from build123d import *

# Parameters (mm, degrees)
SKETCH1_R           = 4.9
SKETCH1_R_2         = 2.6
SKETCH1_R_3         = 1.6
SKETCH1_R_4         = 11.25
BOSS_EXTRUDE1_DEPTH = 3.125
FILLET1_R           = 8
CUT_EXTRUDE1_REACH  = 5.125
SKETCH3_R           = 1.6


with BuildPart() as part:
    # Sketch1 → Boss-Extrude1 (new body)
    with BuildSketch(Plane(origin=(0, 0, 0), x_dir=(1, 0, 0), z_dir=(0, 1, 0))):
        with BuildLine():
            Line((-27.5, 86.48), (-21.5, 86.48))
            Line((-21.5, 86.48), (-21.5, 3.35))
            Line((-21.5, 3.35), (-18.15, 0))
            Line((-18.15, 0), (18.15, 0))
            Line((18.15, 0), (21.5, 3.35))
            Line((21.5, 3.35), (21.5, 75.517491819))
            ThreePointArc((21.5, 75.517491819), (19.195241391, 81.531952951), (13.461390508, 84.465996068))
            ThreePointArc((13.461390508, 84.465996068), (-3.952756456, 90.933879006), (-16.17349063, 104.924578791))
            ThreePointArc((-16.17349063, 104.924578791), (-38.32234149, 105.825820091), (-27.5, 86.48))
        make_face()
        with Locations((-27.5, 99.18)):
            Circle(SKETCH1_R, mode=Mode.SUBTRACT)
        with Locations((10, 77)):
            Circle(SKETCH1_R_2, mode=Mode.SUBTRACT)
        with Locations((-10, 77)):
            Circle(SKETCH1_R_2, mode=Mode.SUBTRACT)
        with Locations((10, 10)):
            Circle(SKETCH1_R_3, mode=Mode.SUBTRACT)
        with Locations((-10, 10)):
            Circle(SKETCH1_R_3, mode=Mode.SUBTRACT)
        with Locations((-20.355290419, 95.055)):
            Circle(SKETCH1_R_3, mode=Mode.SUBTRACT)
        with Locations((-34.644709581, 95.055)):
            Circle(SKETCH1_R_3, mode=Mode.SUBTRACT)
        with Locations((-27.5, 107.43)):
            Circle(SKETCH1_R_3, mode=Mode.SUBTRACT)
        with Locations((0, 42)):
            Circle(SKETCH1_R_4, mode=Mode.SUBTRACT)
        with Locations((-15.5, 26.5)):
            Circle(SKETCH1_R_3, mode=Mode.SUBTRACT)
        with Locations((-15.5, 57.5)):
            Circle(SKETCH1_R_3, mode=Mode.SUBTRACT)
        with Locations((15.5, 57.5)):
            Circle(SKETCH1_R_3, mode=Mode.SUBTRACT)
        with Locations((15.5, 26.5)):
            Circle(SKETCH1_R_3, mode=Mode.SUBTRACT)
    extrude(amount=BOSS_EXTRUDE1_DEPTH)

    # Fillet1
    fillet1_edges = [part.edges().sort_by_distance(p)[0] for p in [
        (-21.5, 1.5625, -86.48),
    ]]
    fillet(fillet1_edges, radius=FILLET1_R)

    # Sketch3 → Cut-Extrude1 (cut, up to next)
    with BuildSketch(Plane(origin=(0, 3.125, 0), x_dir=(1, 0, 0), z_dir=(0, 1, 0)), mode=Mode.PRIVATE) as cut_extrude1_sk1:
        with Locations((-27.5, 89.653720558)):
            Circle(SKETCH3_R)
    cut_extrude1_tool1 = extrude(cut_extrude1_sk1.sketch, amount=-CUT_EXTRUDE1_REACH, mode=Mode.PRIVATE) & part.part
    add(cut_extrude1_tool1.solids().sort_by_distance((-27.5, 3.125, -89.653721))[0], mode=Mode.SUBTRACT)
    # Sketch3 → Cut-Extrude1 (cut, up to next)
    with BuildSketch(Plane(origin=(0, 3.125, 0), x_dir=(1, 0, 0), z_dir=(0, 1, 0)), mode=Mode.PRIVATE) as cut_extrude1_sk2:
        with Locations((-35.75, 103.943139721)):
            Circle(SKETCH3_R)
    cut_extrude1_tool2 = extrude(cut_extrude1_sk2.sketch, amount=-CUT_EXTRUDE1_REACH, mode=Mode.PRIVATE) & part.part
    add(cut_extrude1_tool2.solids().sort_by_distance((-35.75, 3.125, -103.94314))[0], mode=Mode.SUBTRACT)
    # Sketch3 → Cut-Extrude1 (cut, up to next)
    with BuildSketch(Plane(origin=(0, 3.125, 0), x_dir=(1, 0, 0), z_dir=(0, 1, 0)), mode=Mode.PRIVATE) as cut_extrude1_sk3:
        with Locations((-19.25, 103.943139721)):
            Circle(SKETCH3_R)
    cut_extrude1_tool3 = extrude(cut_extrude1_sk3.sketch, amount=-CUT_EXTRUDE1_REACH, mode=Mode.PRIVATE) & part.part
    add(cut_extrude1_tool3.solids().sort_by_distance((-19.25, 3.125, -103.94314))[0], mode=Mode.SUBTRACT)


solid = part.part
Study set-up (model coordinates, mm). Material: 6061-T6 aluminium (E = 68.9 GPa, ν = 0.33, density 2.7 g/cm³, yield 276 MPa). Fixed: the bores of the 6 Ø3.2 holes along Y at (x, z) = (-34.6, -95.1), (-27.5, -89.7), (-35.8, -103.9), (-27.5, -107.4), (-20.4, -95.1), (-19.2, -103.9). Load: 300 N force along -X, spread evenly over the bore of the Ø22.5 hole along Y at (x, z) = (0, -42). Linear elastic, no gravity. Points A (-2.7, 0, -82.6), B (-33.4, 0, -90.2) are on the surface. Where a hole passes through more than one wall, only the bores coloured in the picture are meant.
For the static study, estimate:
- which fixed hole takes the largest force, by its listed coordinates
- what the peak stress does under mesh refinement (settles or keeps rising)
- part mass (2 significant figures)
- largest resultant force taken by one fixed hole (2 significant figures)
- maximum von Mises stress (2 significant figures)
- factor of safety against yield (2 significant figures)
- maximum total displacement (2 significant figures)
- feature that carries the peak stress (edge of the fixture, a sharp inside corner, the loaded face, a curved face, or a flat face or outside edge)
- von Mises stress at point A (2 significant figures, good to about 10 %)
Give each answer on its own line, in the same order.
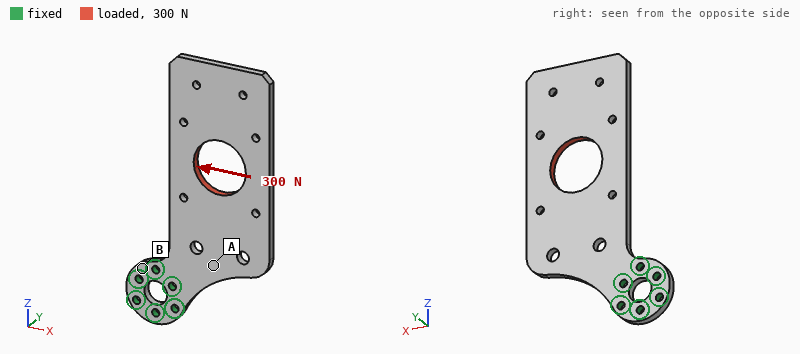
(-27.5, -89.7)
settles
31 g
1.1 kN
130 MPa
2.1
0.25 mm
a curved face
22 MPa
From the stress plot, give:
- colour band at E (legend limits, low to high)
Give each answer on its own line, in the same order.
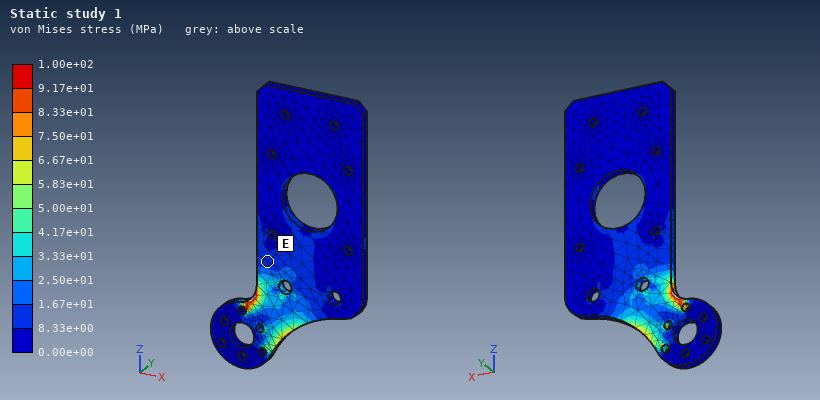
8.33e+00 to 1.67e+01 MPa
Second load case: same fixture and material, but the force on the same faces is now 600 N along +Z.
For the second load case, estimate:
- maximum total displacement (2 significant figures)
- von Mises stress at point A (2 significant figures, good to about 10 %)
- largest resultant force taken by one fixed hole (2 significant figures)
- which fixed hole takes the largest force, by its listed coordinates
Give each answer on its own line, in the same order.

0.17 mm
19 MPa
750 N
(-27.5, -89.7)
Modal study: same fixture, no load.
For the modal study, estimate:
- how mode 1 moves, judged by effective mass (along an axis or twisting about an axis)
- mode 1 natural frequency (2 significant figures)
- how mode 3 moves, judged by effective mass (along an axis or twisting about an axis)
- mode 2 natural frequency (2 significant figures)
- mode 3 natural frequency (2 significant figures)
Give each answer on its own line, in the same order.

along Y
210 Hz
along X
800 Hz
1300 Hz
